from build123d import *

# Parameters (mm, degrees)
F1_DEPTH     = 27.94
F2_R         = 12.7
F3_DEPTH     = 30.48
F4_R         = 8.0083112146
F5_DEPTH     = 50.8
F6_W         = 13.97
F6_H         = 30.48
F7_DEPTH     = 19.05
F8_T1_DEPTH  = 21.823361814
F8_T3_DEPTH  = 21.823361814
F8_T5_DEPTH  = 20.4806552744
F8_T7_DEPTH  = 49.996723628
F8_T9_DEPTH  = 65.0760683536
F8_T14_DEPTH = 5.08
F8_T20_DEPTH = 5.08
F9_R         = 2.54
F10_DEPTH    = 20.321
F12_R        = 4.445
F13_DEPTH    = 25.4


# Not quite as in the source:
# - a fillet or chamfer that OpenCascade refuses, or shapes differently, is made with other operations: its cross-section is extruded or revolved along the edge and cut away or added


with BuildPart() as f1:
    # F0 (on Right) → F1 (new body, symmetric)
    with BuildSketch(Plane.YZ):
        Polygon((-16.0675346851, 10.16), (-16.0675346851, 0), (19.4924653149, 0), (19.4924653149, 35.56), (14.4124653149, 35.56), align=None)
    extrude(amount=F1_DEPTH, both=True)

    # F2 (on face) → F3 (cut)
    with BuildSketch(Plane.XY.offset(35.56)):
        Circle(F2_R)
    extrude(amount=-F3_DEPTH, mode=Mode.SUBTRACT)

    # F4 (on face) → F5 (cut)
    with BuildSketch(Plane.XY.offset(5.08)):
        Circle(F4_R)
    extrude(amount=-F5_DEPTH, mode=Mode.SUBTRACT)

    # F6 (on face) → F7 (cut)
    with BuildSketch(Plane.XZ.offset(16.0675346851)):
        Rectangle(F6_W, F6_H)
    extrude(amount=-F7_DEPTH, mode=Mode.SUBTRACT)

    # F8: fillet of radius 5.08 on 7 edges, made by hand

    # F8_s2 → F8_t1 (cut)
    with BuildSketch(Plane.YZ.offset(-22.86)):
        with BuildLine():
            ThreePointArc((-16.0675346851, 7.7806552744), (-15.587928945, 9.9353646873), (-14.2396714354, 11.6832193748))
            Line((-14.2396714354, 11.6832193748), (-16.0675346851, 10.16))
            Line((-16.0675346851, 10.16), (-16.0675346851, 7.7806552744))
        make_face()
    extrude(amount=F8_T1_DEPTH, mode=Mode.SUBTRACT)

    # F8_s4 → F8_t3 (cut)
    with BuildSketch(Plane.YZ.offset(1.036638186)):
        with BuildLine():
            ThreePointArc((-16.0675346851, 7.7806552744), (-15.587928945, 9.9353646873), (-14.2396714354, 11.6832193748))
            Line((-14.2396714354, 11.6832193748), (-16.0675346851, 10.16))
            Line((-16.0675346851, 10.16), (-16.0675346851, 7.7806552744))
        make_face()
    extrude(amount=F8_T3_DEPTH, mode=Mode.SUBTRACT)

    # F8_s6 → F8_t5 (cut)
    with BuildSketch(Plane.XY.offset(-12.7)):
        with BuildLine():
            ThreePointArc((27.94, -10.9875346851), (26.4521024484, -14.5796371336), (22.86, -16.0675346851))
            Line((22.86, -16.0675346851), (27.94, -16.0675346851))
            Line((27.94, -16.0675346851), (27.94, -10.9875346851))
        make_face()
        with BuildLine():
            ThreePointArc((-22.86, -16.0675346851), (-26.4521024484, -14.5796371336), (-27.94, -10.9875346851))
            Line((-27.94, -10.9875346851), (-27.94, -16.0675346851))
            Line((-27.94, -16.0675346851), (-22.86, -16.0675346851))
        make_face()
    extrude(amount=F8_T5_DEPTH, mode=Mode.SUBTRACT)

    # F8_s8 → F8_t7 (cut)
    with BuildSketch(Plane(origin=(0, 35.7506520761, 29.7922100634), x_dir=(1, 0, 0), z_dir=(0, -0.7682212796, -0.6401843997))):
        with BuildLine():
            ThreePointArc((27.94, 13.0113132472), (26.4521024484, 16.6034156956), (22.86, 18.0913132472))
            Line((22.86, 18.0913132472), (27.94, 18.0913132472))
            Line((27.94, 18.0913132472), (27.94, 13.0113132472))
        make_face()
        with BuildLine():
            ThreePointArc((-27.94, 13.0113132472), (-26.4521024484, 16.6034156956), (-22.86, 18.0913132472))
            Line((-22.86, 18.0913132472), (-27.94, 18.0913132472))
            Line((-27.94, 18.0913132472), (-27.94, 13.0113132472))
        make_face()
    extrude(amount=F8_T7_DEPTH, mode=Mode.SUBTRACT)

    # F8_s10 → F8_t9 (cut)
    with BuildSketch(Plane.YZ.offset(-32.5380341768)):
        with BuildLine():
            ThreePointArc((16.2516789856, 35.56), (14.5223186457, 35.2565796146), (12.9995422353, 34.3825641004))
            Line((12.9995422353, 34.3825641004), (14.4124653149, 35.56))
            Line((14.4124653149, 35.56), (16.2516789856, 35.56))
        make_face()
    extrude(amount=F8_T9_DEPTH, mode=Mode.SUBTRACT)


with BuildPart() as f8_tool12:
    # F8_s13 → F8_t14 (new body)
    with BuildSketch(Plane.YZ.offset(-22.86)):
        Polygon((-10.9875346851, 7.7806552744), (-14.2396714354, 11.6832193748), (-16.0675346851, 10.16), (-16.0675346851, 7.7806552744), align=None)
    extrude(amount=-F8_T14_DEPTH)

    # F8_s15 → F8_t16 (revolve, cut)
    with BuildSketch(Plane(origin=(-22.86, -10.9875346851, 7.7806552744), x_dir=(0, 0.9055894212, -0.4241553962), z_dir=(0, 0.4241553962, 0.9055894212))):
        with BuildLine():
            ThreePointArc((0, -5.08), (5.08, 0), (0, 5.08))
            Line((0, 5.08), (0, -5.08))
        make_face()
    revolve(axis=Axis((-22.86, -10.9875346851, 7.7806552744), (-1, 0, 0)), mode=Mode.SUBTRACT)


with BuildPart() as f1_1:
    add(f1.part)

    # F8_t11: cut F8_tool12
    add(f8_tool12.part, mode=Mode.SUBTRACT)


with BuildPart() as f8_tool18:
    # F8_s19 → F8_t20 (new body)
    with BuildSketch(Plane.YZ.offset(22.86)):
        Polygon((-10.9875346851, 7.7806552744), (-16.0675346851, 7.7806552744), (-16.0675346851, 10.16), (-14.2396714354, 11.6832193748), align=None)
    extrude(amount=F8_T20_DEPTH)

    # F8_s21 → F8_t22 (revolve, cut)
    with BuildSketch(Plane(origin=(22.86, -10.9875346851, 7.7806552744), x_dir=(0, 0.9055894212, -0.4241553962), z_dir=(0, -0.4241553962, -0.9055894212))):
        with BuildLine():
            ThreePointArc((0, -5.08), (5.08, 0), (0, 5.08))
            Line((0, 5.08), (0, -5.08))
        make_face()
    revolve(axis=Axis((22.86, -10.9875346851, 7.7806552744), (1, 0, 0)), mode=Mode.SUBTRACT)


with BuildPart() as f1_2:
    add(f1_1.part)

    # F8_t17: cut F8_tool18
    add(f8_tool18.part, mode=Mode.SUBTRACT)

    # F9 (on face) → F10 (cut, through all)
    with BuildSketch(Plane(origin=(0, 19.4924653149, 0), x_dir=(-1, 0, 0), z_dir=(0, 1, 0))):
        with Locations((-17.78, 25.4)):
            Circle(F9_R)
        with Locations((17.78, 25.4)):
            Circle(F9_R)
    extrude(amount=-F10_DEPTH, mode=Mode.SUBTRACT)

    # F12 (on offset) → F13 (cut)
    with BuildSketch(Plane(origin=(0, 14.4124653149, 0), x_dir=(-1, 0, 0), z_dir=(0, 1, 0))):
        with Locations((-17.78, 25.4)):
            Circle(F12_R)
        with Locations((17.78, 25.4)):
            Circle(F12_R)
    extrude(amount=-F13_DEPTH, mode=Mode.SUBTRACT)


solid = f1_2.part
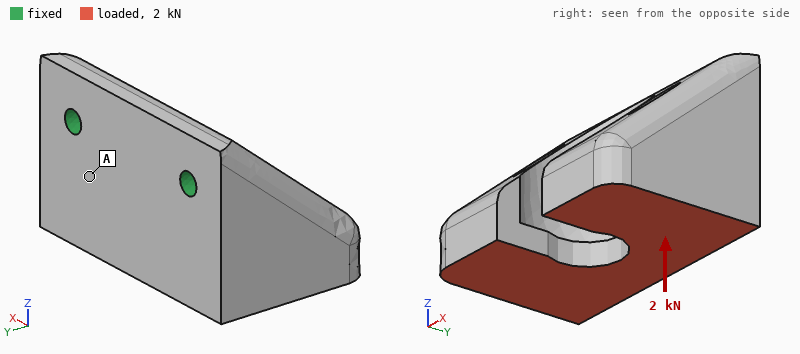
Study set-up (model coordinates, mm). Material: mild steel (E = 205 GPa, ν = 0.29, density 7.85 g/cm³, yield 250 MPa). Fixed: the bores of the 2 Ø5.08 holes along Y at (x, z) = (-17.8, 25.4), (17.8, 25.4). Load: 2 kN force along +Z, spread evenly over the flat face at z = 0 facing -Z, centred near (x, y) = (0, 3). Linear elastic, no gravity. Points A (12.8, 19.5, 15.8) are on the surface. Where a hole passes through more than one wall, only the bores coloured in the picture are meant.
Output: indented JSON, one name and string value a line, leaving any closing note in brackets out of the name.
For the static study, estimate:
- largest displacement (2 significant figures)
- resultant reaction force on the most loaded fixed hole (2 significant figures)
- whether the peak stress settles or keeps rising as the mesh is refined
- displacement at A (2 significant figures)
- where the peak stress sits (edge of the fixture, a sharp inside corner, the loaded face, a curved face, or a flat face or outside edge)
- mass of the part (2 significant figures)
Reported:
{
  "largest displacement": "27 µm",
  "resultant reaction force on the most loaded fixed hole": "1.0 kN",
  "whether the peak stress settles or keeps rising as the mesh is refined": "keeps rising",
  "displacement at A": "5.5 µm",
  "where the peak stress sits": "edge of the fixture",
  "mass of the part": "280 g"
}
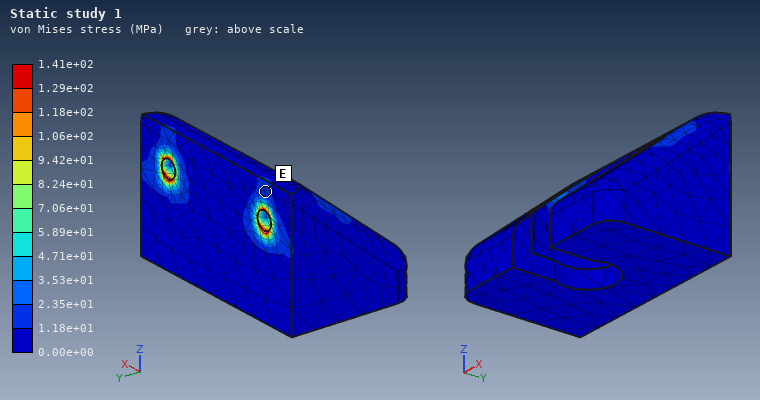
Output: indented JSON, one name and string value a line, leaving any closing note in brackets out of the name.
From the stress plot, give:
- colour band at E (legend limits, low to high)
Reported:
{
  "colour band at E": "1.18e+01 to 2.35e+01 MPa"
}
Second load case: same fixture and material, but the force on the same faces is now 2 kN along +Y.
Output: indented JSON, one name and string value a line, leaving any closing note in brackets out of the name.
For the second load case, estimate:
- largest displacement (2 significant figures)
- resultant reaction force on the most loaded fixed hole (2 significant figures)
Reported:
{
  "largest displacement": "49 µm",
  "resultant reaction force on the most loaded fixed hole": "1.0 kN"
}
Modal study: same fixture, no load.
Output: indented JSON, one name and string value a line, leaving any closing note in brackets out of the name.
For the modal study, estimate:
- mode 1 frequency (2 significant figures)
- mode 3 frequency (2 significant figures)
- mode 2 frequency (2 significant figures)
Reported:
{
  "mode 1 frequency": "3100 Hz",
  "mode 3 frequency": "6800 Hz",
  "mode 2 frequency": "5400 Hz"
}
